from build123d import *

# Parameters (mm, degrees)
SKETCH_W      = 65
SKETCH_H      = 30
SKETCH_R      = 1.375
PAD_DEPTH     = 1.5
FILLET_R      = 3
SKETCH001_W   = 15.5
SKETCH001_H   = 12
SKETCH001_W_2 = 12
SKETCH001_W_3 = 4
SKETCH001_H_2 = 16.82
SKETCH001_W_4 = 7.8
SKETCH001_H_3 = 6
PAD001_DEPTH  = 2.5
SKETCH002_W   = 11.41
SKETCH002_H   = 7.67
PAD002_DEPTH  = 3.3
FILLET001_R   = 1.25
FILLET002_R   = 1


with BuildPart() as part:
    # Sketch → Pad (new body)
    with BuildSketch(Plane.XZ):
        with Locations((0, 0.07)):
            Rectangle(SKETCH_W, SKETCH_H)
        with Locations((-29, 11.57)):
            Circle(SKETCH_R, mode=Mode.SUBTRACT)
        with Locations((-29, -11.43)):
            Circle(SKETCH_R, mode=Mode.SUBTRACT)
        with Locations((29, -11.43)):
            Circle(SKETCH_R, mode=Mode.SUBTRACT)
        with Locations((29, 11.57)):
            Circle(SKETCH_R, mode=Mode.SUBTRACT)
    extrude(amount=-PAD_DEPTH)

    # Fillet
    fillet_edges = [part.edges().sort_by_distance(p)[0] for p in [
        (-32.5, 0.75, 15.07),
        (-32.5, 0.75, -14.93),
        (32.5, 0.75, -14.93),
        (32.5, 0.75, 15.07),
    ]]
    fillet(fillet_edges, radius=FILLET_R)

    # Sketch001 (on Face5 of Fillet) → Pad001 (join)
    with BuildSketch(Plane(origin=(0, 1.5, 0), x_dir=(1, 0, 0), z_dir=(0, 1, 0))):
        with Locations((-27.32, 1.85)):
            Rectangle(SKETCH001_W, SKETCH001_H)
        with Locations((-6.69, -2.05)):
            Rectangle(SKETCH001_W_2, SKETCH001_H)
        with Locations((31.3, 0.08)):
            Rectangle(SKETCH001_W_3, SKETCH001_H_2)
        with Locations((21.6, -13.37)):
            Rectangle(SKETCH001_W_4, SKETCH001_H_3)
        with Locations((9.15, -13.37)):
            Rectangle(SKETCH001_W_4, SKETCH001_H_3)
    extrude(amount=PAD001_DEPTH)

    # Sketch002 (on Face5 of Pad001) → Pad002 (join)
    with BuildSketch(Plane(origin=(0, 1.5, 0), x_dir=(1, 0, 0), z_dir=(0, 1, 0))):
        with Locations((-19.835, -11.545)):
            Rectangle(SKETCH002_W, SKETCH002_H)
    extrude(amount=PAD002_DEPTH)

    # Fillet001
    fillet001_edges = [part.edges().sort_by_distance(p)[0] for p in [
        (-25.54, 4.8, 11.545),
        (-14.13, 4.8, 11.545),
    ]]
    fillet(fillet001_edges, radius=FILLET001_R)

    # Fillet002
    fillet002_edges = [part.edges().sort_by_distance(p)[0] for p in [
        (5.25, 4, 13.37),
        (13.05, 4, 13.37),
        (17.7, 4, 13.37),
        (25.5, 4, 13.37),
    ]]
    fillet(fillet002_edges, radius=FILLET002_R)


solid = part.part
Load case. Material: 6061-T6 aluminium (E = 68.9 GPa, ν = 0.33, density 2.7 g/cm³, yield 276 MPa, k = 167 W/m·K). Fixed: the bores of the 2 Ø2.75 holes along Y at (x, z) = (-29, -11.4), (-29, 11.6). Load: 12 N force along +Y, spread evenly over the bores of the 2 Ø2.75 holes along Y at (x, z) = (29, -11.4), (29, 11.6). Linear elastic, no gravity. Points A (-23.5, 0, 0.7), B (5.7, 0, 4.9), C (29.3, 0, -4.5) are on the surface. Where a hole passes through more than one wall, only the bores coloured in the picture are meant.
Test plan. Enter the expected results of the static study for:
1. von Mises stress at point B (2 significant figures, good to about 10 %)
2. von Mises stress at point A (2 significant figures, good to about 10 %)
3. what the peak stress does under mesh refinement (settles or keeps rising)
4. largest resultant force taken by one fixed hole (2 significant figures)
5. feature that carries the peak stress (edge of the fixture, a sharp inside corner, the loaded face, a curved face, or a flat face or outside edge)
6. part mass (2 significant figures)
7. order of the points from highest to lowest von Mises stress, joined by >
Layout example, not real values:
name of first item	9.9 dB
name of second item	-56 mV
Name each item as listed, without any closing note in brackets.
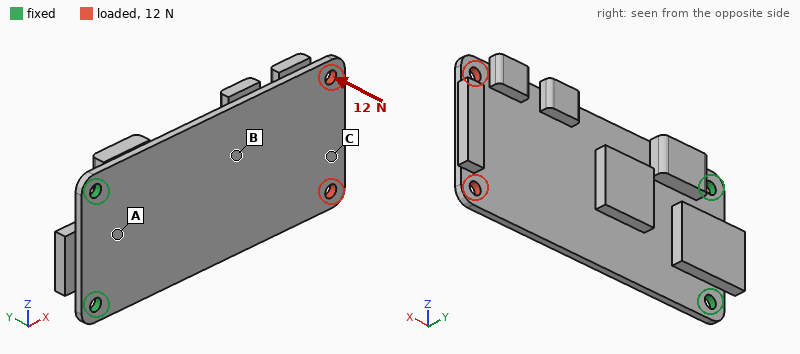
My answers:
von Mises stress at point B	20 MPa
von Mises stress at point A	10 MPa
what the peak stress does under mesh refinement	keeps rising
largest resultant force taken by one fixed hole	9.4 N
feature that carries the peak stress	edge of the fixture
part mass	12 g
order of the points from highest to lowest von Mises stress, joined by >	B > A > C
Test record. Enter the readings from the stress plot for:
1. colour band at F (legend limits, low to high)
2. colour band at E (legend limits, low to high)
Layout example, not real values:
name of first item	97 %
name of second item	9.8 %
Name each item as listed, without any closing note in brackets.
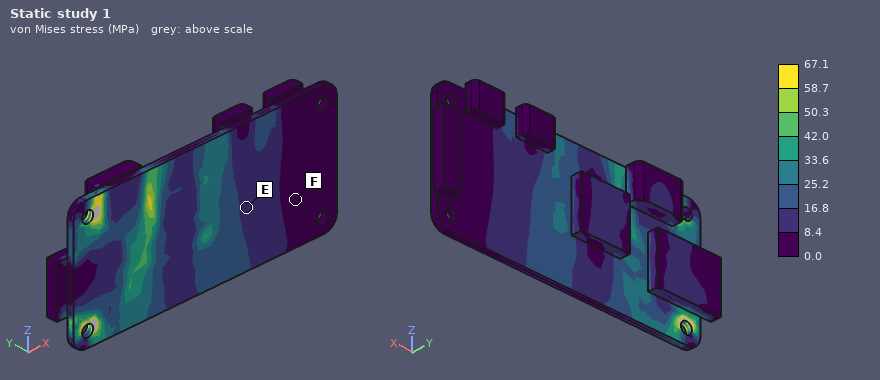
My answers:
colour band at F	0.0 to 8.4 MPa
colour band at E	8.4 to 16.8 MPa
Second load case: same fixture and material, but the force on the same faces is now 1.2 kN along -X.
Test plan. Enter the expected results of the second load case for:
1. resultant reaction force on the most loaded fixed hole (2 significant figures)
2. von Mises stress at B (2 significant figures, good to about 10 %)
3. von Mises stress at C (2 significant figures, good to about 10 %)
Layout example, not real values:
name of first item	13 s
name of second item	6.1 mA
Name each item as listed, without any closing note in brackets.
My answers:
resultant reaction force on the most loaded fixed hole	610 N
von Mises stress at B	27 MPa
von Mises stress at C	16 MPa
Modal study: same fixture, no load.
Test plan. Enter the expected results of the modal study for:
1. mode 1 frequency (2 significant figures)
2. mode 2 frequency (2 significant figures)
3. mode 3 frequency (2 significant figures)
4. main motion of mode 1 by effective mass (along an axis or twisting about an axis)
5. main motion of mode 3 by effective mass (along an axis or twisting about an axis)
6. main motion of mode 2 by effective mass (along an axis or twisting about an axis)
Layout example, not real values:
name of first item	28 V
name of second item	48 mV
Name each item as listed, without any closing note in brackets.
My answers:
mode 1 frequency	390 Hz
mode 2 frequency	1800 Hz
mode 3 frequency	2000 Hz
main motion of mode 1 by effective mass	along Y
main motion of mode 3 by effective mass	along Y
main motion of mode 2 by effective mass	twisting about X
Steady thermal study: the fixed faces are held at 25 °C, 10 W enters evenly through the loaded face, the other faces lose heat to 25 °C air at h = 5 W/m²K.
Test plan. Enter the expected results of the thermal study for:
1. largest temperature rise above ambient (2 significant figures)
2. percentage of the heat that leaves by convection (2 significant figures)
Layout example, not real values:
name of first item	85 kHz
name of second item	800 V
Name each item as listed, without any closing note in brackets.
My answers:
largest temperature rise above ambient	72 K
percentage of the heat that leaves by convection	7.7 %
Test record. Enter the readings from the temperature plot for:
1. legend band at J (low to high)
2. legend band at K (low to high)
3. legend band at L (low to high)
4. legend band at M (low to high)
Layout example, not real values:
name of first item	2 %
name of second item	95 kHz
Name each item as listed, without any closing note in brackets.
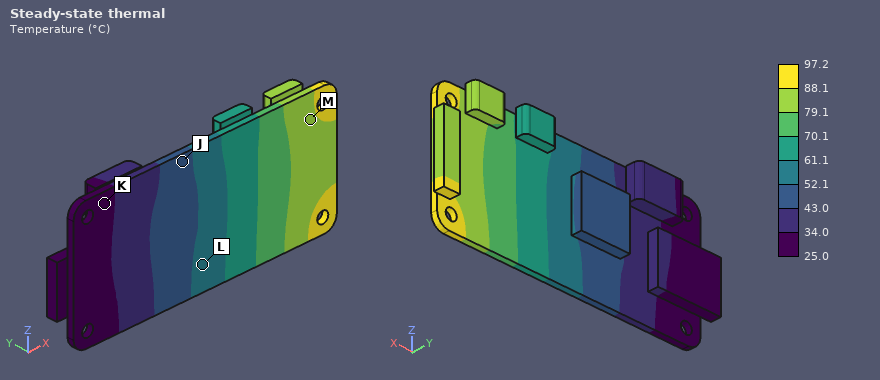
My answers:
legend band at J	43.0 to 52.1 °C
legend band at K	25.0 to 34.0 °C
legend band at L	52.1 to 61.1 °C
legend band at M	79.1 to 88.1 °C
